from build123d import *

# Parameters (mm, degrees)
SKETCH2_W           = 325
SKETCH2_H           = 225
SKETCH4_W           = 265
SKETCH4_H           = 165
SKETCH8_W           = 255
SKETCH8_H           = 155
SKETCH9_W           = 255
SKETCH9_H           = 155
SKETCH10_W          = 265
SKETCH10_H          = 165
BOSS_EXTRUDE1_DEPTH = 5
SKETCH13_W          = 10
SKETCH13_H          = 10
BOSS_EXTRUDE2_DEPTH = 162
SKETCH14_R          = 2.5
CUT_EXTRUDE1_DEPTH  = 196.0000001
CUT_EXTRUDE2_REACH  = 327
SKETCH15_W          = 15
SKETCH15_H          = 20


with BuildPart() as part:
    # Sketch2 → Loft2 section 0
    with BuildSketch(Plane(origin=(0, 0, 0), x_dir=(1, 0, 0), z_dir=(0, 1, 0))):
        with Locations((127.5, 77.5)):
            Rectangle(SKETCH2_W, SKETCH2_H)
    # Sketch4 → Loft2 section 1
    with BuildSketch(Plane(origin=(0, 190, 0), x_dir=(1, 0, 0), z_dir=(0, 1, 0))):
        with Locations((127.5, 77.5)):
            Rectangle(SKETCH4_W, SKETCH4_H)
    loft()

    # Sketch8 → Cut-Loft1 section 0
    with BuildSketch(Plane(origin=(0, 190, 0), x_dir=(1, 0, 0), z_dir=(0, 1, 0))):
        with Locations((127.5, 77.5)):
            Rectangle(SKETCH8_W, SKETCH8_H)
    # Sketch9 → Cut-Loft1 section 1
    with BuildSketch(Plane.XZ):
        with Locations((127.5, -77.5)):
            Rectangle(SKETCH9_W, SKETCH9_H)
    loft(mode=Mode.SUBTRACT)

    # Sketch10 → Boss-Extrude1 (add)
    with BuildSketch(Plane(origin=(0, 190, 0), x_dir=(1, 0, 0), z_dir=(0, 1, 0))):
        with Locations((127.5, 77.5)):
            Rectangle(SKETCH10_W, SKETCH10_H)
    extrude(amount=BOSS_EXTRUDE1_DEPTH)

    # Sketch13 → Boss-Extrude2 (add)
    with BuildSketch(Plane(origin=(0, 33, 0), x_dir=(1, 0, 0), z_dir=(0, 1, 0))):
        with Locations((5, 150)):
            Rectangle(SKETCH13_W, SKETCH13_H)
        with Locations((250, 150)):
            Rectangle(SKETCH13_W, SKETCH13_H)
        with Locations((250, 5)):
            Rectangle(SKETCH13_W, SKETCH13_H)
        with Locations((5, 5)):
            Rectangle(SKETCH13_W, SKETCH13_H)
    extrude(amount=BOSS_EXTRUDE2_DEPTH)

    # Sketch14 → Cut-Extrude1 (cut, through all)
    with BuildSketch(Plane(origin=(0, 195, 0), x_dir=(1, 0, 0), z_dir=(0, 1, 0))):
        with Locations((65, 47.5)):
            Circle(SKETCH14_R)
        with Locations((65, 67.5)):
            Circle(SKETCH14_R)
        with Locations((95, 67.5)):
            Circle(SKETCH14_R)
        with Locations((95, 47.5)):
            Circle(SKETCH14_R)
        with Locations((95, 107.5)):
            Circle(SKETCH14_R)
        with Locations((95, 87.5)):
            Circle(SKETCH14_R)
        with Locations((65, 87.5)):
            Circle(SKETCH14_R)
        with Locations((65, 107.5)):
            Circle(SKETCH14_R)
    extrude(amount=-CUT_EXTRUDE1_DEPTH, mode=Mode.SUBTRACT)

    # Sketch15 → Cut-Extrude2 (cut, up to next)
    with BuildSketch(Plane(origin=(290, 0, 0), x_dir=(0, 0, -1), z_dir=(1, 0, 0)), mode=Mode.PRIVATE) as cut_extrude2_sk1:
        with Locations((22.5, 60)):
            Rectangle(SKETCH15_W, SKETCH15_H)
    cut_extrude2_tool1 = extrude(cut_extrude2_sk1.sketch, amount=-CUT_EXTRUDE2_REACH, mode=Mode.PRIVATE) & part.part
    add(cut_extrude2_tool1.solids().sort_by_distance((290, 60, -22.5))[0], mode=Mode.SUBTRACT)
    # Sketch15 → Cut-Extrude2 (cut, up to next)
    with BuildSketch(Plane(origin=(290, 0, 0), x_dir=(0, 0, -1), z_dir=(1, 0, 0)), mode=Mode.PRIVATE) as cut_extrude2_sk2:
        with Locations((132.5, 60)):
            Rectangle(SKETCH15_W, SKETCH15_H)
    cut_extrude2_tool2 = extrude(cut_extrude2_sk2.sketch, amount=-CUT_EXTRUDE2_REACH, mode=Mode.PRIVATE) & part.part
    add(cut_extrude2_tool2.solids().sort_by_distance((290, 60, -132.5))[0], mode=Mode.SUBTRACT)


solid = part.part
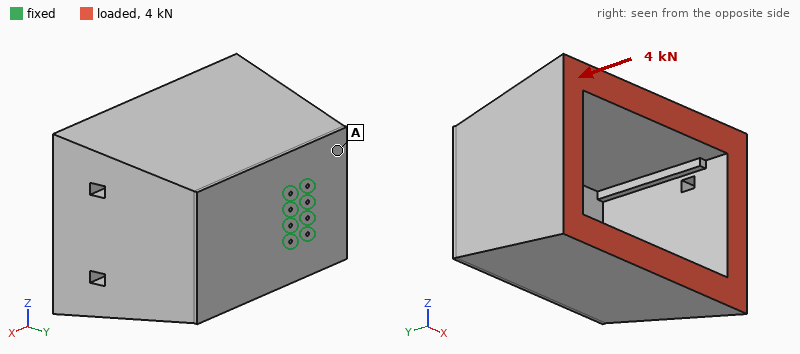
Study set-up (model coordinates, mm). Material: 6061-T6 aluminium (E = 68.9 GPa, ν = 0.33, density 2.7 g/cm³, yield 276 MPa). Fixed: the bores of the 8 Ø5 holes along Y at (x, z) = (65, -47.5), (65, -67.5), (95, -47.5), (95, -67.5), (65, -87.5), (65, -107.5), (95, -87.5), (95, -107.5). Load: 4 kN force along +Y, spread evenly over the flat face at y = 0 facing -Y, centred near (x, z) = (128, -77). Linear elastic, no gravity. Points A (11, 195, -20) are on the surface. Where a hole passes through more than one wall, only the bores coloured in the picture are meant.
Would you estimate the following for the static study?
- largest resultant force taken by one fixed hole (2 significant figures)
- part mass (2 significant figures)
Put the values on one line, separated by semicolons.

3.1 kN; 10 kg
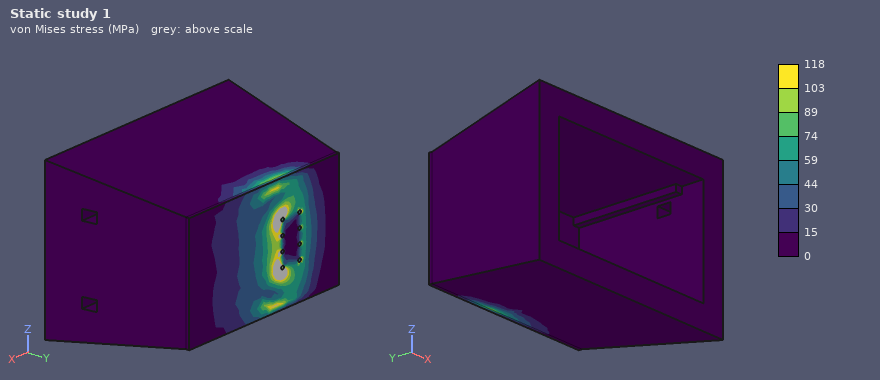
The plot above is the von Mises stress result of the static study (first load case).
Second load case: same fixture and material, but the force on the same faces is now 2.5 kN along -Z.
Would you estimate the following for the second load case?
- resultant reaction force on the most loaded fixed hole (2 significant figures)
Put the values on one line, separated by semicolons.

3.3 kN
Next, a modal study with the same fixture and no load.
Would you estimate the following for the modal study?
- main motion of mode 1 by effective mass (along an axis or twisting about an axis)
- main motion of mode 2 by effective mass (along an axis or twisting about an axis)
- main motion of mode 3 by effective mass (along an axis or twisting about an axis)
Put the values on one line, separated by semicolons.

along X; along Z; along Y
